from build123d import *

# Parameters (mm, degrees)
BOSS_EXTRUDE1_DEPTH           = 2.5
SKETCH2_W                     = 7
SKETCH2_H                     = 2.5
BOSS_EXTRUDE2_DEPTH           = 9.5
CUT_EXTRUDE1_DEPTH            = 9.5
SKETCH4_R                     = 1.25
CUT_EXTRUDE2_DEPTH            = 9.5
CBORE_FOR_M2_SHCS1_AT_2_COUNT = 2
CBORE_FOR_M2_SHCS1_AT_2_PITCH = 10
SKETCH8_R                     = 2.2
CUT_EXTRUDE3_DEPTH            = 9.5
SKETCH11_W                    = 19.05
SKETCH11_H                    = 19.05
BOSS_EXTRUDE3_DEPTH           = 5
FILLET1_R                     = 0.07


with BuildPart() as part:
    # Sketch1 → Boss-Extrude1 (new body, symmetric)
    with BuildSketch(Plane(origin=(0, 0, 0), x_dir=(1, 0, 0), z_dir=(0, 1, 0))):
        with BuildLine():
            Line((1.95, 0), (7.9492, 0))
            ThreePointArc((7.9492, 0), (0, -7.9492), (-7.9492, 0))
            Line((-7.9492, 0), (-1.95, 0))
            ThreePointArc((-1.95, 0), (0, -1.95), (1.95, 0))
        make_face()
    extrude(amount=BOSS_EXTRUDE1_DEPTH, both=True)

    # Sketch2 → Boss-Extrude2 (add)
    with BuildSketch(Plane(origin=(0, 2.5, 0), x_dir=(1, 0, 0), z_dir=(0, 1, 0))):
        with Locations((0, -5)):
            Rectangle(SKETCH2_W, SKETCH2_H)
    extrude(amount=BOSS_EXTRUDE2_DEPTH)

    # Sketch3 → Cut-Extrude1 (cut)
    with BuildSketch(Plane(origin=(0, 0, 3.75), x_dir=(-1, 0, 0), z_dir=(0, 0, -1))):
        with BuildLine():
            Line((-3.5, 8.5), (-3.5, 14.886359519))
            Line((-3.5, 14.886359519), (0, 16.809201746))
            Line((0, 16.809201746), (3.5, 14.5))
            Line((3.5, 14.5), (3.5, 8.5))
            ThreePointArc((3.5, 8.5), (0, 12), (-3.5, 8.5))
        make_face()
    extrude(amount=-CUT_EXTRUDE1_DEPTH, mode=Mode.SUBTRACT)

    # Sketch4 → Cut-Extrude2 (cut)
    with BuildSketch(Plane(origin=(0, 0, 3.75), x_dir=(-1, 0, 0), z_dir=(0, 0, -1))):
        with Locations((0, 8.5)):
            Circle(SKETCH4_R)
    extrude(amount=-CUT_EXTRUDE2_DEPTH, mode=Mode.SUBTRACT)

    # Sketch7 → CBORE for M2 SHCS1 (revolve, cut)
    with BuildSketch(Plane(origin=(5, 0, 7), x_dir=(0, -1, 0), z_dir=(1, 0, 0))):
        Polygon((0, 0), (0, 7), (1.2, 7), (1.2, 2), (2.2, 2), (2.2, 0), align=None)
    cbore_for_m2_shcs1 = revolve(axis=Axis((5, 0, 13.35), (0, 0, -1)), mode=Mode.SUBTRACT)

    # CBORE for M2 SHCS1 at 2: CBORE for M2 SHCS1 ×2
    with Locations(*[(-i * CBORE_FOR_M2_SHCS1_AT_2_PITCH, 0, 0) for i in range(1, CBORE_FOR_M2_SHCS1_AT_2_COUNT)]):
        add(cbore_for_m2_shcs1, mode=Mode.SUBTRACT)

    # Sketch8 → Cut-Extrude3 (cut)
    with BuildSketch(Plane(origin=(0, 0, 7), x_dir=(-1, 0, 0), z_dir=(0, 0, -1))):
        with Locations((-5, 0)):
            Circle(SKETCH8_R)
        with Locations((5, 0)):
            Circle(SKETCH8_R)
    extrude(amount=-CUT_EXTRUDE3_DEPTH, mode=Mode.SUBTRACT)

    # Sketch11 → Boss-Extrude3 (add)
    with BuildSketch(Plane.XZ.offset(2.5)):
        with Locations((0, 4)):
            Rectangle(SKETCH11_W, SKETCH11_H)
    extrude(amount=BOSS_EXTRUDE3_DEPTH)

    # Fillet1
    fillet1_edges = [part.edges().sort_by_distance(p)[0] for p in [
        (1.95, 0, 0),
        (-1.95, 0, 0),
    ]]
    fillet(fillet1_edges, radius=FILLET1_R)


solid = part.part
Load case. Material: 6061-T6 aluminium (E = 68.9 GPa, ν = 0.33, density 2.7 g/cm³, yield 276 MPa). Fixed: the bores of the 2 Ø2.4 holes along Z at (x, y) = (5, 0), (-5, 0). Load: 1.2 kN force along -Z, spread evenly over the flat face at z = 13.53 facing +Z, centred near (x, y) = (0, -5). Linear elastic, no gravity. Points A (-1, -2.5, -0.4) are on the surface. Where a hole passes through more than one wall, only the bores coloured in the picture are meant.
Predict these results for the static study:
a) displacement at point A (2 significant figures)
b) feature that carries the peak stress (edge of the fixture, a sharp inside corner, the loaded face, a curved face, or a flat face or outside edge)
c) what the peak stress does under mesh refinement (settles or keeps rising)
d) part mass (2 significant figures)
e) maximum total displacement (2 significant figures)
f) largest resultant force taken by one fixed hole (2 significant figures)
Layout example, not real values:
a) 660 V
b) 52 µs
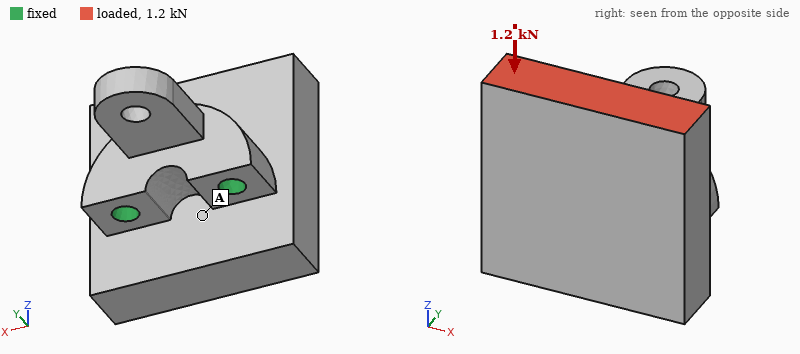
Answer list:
a) 5.0 µm
b) edge of the fixture
c) keeps rising
d) 6.3 g
e) 20 µm
f) 600 N
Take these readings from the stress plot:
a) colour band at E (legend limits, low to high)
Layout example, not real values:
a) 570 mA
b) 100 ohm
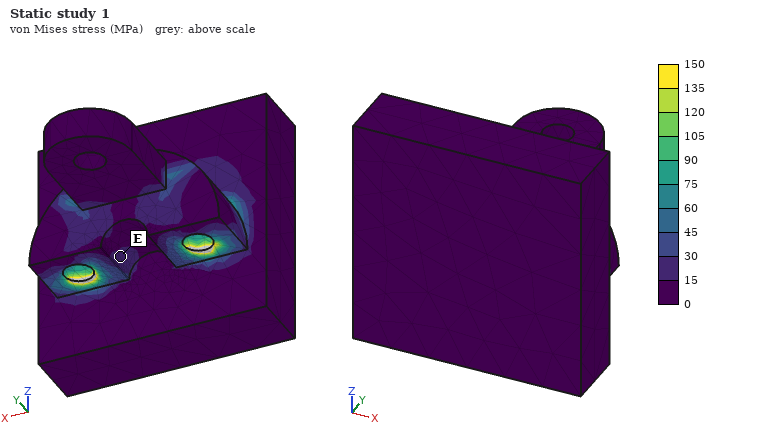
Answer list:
a) 15 to 30 MPa
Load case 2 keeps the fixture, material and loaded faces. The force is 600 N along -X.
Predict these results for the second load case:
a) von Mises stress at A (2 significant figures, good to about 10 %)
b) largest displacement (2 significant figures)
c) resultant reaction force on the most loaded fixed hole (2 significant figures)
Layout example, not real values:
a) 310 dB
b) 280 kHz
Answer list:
a) 10 MPa
b) 13 µm
c) 690 N
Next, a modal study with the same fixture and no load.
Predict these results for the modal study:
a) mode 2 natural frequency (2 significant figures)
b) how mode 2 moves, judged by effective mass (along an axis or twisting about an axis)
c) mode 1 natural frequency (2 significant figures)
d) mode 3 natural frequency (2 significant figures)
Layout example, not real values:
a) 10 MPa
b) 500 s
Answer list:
a) 23 kHz
b) along Z
c) 17 kHz
d) 29 kHz
